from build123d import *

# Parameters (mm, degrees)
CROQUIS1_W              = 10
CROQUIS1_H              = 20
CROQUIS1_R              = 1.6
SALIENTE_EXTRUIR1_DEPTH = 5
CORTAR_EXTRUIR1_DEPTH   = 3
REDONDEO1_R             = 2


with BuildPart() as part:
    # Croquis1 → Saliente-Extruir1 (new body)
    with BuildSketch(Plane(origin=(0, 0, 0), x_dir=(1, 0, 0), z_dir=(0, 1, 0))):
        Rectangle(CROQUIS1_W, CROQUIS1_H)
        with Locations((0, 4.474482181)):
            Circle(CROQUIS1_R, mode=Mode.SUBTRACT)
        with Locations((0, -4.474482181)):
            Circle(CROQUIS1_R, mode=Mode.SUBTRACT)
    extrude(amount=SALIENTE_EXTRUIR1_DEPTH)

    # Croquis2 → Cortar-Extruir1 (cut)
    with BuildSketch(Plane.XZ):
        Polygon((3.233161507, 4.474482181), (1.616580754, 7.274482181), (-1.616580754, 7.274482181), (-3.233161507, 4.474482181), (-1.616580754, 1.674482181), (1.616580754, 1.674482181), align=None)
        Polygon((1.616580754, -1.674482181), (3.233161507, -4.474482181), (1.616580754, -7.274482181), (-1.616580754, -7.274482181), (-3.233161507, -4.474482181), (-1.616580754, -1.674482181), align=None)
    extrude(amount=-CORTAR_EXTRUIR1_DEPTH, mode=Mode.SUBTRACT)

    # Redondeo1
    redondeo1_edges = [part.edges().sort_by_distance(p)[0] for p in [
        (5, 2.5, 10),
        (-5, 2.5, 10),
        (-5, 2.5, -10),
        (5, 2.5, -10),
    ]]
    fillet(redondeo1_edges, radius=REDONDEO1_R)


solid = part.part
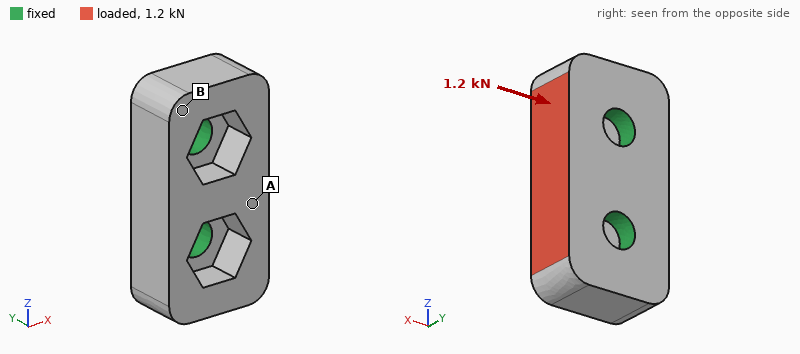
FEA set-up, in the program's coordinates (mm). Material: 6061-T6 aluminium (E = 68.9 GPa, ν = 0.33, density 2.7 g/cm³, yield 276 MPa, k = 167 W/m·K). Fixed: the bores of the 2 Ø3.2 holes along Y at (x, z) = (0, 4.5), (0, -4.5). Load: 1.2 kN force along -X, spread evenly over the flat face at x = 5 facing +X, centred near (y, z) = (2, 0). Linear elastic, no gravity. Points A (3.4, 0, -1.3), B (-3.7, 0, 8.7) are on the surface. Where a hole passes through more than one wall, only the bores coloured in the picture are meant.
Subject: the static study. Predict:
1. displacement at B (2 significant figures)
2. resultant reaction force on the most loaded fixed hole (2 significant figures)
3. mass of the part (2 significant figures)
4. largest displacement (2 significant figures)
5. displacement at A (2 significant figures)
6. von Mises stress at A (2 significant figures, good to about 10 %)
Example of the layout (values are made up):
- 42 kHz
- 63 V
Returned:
- 7.0 µm
- 600 N
- 2.1 g
- 11 µm
- 8.6 µm
- 33 MPa
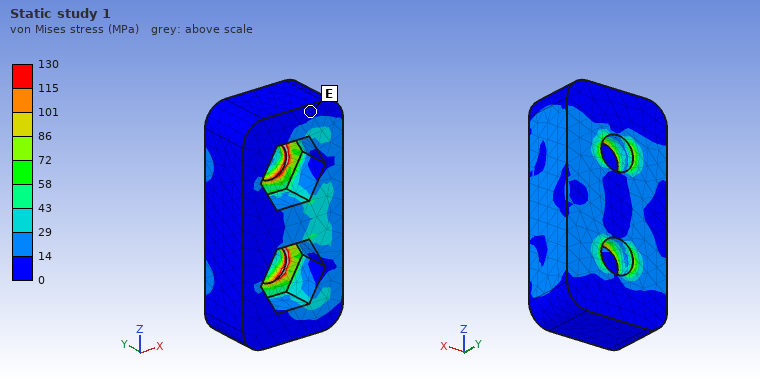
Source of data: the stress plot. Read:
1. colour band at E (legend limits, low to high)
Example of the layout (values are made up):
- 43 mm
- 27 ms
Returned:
- 0 to 14 MPa
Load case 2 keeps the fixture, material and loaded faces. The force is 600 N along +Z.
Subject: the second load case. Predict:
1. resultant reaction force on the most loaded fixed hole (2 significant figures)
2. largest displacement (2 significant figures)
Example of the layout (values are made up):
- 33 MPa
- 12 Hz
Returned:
- 390 N
- 4.1 µm
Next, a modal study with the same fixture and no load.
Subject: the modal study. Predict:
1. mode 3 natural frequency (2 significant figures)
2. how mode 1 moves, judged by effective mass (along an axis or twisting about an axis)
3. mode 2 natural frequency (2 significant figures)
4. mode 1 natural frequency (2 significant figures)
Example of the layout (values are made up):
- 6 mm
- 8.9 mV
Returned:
- 53 kHz
- along X
- 52 kHz
- 40 kHz
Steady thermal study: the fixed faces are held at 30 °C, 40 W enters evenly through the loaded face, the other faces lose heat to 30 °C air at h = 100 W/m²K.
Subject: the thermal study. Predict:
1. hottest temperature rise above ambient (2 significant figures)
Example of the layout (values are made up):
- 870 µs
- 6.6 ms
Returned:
- 22 K
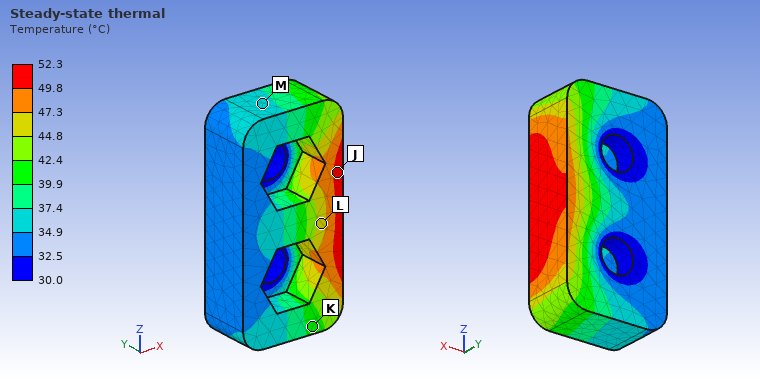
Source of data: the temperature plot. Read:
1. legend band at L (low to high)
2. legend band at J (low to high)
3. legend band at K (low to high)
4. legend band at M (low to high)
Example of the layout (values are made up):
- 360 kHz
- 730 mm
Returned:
- 44.8 to 47.3 °C
- 49.8 to 52.3 °C
- 39.9 to 42.4 °C
- 34.9 to 37.4 °C
